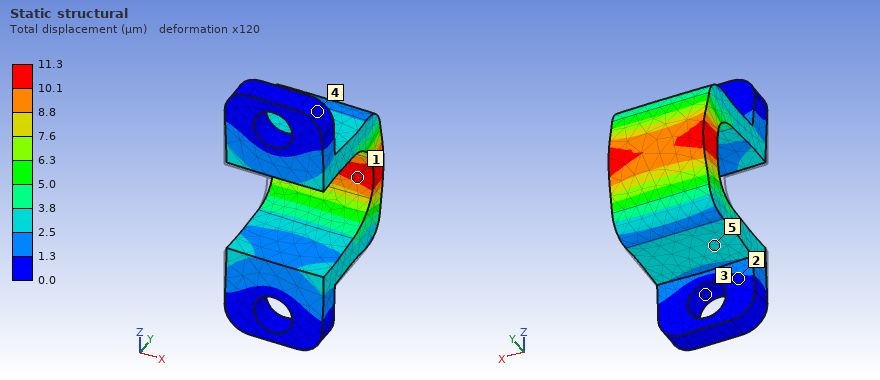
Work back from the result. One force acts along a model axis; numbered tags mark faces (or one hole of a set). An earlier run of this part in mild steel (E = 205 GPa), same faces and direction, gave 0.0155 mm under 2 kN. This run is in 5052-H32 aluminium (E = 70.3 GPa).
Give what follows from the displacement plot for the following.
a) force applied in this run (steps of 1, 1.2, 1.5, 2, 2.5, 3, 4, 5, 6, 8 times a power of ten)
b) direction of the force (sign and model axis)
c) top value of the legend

500 N
+Y
11.3 µm
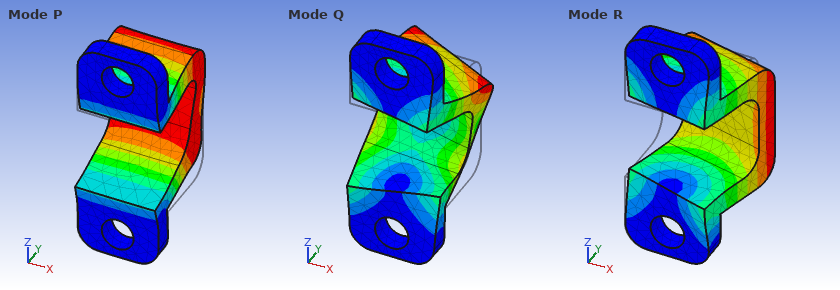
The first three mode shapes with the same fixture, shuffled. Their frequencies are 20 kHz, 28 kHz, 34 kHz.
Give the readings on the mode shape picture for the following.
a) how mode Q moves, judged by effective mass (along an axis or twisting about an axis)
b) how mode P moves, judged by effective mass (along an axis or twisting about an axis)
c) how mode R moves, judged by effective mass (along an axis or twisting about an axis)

twisting about Y
along Z
along X
